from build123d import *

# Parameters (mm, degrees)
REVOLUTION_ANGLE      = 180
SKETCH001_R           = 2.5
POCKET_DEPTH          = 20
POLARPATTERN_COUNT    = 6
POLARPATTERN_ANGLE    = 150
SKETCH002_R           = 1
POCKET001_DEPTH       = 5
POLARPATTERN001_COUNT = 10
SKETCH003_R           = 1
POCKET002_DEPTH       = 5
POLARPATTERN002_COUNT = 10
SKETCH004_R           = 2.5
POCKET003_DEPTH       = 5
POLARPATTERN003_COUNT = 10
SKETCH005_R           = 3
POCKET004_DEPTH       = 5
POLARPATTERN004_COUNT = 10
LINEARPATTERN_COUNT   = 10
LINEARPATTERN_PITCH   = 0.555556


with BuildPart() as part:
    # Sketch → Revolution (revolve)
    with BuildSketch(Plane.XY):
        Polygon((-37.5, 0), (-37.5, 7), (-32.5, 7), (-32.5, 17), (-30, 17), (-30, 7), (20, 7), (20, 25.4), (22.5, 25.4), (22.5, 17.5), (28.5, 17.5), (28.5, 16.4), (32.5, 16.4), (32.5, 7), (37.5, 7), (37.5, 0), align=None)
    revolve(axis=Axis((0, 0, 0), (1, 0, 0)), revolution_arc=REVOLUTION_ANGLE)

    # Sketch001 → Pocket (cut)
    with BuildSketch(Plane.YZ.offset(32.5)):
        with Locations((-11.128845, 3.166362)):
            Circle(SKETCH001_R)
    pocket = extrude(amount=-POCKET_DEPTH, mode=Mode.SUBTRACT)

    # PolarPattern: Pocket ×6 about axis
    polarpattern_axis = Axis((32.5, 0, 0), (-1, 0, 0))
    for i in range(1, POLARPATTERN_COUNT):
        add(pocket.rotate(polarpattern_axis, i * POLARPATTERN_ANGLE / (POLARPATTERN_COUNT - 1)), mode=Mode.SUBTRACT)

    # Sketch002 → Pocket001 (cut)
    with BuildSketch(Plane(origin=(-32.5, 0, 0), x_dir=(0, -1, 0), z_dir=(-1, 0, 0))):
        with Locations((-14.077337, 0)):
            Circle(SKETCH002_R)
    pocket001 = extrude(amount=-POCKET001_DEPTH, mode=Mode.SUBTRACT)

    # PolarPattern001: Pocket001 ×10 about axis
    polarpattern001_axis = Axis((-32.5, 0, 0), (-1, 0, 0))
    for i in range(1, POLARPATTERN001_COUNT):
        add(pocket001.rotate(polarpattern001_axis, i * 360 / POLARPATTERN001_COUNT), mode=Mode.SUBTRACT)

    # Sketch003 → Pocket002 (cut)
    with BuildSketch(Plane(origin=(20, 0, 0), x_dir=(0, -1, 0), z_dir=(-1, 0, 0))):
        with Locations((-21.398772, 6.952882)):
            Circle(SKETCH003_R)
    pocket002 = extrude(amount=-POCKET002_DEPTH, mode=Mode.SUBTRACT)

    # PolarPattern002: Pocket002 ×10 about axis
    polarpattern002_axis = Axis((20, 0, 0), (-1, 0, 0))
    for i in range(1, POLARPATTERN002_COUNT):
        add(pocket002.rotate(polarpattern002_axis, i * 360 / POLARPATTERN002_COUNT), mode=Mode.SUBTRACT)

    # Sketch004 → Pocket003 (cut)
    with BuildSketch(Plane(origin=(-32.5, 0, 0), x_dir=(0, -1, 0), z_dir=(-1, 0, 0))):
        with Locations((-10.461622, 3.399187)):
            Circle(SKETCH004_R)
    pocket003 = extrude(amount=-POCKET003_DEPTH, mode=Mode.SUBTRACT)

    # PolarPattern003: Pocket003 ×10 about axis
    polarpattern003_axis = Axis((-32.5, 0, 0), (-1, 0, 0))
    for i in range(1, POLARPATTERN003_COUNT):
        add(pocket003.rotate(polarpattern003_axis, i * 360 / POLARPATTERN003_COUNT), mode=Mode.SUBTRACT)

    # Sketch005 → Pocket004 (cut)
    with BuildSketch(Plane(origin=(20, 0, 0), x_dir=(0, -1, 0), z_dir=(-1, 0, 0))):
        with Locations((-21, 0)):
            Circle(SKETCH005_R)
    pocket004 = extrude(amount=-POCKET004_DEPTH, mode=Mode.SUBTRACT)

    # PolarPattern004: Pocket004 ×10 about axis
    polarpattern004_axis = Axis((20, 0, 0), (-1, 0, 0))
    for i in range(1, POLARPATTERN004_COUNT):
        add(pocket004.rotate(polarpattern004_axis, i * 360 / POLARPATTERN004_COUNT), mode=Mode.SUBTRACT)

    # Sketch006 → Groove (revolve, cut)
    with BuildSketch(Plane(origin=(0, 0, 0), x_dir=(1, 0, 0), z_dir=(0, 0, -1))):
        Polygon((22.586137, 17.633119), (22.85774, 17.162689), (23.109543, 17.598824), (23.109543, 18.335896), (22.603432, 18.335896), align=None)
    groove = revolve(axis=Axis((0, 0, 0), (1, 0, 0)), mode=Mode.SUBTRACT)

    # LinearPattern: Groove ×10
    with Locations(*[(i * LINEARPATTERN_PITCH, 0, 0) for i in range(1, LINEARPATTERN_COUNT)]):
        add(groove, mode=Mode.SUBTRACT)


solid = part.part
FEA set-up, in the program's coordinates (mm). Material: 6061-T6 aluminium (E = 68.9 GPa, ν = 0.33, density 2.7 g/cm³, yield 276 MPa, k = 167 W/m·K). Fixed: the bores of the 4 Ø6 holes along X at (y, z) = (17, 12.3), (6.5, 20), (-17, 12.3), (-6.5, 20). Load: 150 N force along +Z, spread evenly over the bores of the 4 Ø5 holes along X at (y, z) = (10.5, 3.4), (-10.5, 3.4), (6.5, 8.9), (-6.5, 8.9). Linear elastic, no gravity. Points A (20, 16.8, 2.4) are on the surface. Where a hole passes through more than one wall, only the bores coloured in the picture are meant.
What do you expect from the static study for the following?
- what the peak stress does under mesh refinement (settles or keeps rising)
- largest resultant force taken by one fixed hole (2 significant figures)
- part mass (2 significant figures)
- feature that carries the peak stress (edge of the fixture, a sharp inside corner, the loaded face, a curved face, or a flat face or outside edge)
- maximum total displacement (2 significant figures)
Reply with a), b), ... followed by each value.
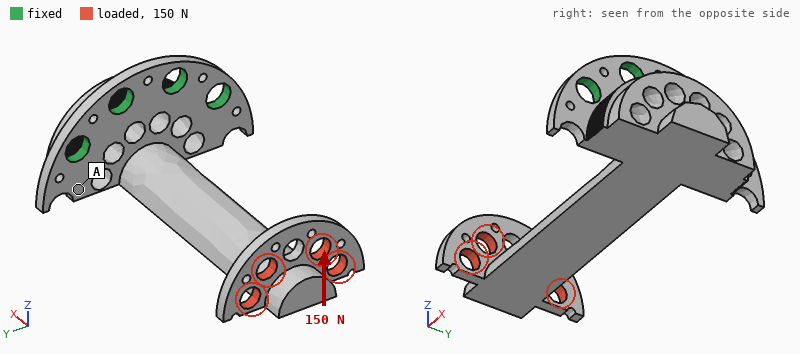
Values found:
a) keeps rising
b) 500 N
c) 29 g
d) edge of the fixture
e) 0.63 mm
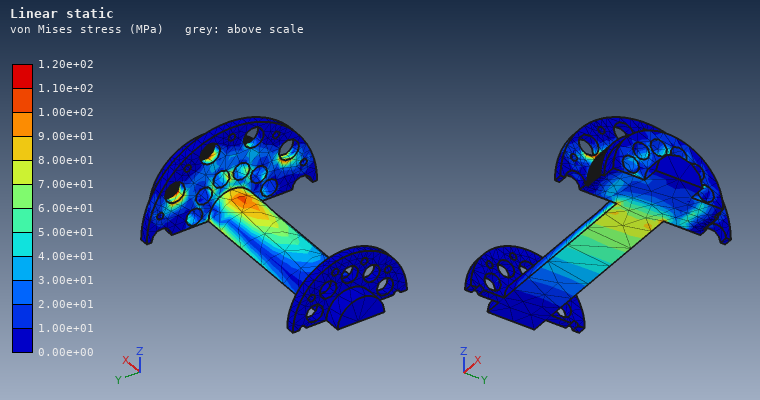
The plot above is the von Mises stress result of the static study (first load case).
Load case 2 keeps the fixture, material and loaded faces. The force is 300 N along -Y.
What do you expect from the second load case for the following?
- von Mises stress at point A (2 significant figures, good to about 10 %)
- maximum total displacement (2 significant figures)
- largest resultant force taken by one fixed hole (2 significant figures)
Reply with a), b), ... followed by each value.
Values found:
a) 16 MPa
b) 0.39 mm
c) 510 N
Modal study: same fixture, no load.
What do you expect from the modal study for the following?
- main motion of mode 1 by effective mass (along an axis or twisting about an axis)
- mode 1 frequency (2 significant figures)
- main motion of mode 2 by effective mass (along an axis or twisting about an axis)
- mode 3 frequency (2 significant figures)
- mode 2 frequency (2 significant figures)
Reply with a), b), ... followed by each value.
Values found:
a) along Z
b) 1100 Hz
c) along Y
d) 5200 Hz
e) 1900 Hz
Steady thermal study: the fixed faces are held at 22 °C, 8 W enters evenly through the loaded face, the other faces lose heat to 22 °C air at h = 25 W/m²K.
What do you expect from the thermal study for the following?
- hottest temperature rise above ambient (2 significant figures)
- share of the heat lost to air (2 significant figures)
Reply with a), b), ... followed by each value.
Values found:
a) 38 K
b) 24 %
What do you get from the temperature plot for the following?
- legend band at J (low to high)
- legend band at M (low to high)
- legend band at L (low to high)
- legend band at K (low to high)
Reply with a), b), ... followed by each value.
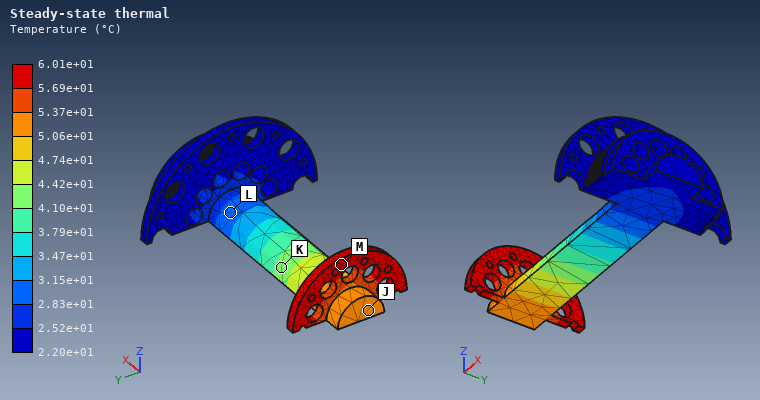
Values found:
a) 5.06e+01 to 5.37e+01 °C
b) 5.69e+01 to 6.01e+01 °C
c) 2.83e+01 to 3.15e+01 °C
d) 4.10e+01 to 4.42e+01 °C
